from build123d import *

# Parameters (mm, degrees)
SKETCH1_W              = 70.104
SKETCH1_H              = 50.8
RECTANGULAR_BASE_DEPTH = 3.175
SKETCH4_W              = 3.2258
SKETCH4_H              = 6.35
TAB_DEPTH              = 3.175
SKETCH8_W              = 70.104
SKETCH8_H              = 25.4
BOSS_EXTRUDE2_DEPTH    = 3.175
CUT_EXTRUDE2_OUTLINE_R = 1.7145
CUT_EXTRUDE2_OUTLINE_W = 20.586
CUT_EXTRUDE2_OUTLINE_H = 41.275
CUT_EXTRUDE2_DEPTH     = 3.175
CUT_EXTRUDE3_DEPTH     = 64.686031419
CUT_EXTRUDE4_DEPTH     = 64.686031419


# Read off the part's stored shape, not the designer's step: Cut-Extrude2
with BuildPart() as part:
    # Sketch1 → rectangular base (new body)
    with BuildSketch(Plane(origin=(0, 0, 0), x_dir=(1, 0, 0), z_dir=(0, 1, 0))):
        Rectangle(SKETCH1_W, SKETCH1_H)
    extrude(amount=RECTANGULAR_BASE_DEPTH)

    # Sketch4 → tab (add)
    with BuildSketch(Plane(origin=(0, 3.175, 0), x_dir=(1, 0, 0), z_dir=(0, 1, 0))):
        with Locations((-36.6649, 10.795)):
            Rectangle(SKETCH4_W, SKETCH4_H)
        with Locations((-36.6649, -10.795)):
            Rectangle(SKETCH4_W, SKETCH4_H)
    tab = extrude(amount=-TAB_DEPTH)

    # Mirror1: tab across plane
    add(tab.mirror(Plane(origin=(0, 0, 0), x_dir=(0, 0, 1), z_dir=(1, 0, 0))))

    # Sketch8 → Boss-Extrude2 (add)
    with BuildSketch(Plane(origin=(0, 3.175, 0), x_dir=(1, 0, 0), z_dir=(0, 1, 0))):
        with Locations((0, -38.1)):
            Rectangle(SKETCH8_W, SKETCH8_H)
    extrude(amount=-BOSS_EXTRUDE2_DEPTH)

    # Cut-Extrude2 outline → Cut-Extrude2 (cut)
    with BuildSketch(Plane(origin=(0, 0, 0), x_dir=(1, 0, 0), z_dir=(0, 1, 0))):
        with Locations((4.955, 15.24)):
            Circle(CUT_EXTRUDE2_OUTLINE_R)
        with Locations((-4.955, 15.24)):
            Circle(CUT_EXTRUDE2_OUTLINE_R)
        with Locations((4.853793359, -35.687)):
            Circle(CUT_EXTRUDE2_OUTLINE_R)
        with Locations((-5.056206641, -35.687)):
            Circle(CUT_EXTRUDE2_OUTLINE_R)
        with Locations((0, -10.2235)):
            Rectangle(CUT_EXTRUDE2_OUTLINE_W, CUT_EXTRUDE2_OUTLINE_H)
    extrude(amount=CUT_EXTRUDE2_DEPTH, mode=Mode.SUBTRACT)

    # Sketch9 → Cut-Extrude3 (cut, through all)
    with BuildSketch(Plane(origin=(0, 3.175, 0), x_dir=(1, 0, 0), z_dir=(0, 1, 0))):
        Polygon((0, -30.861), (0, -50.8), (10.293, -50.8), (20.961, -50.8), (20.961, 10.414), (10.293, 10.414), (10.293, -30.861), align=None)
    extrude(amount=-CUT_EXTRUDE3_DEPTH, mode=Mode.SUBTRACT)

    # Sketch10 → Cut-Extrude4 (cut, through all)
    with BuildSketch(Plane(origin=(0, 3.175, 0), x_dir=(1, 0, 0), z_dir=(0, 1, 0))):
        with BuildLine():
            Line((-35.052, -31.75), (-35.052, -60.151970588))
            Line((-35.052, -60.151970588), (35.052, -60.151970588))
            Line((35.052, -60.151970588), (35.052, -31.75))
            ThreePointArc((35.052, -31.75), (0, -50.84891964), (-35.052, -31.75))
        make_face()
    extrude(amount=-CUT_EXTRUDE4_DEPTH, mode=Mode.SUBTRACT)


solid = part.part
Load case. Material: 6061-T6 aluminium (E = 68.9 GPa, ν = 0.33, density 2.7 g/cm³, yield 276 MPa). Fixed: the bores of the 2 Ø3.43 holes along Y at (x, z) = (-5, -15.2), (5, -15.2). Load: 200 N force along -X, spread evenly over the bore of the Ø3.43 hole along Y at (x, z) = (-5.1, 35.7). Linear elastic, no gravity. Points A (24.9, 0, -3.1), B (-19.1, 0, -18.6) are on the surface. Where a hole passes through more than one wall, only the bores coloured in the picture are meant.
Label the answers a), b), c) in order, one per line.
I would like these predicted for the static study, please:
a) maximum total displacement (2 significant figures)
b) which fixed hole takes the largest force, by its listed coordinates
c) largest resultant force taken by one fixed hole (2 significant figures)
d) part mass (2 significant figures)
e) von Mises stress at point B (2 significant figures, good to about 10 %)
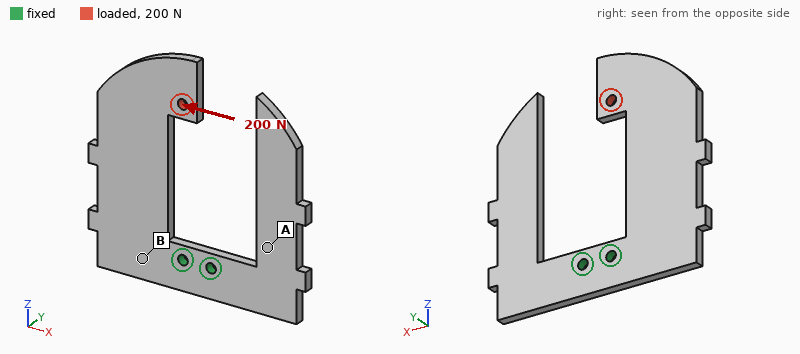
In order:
a) 0.27 mm
b) (-5, -15.2)
c) 830 N
d) 29 g
e) 29 MPa
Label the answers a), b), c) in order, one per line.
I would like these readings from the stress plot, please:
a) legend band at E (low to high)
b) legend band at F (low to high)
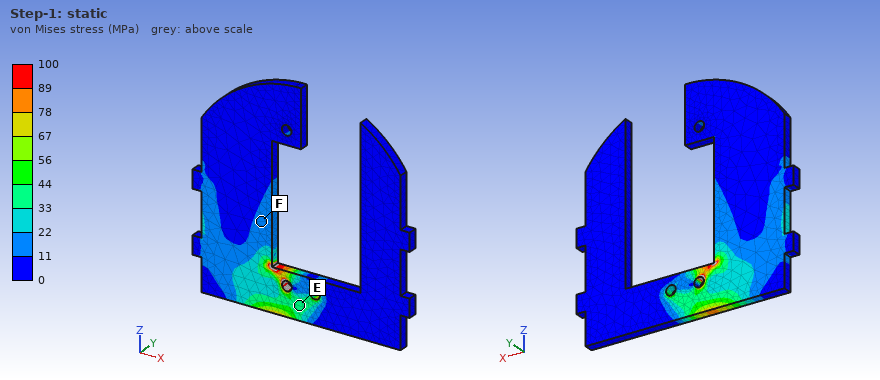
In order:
a) 33 to 44 MPa
b) 11 to 22 MPa
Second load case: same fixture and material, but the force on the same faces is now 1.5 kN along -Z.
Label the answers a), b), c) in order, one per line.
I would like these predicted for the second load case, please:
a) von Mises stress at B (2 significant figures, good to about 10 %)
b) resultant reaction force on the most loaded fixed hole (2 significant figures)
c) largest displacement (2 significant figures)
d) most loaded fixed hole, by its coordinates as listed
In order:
a) 31 MPa
b) 1.4 kN
c) 0.36 mm
d) (-5, -15.2)
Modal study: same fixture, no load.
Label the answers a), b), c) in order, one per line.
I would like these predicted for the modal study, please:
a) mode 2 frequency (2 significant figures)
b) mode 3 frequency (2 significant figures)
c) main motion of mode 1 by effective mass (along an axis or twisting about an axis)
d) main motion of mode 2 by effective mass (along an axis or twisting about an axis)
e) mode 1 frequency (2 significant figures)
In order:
a) 570 Hz
b) 1300 Hz
c) along Y
d) along Y
e) 450 Hz
